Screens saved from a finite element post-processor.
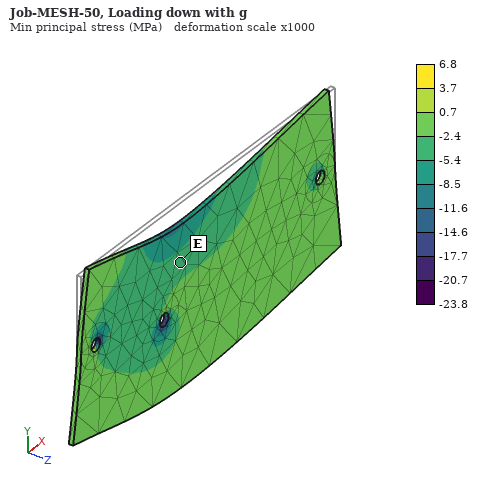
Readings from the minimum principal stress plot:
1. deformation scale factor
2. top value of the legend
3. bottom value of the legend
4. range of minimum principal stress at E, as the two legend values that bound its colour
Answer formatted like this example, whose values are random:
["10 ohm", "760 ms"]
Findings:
["1000", "6.8 MPa", "-23.8 MPa", "-5.4 to -2.4 MPa"]
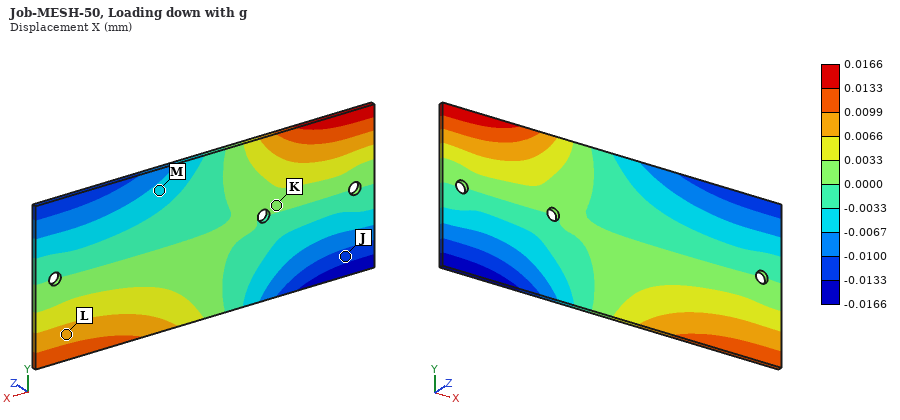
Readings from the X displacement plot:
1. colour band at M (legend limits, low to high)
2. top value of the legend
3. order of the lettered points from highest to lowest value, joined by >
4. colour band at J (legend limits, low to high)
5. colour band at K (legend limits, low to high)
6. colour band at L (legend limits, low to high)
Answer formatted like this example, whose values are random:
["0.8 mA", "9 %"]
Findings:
["-0.0067 to -0.0033 mm", "0.0166 mm", "L > K > M > J", "-0.0133 to -0.0100 mm", "0.0000 to 0.0033 mm", "0.0066 to 0.0099 mm"]
